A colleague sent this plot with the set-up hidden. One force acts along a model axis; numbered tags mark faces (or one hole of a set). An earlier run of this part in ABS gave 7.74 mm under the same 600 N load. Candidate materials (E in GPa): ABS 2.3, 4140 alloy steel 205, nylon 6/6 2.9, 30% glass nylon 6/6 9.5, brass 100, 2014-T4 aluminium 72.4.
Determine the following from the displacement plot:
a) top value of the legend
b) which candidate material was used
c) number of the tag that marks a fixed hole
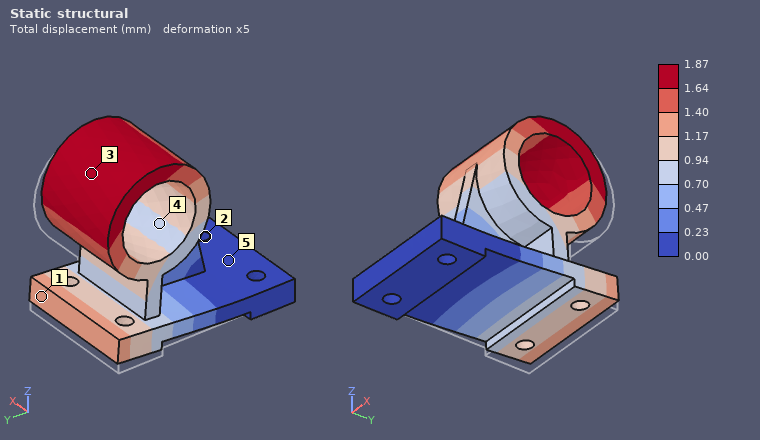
1.87 mm
30% glass nylon 6/6
2
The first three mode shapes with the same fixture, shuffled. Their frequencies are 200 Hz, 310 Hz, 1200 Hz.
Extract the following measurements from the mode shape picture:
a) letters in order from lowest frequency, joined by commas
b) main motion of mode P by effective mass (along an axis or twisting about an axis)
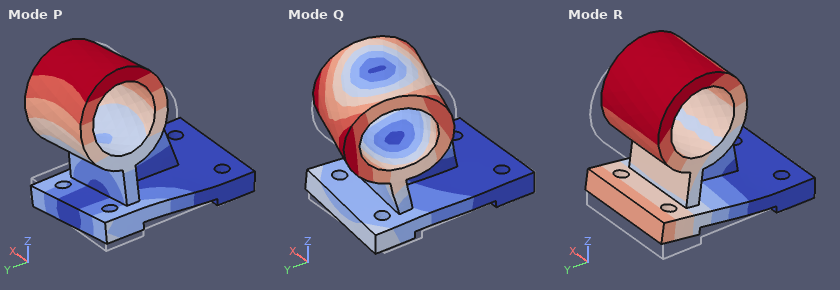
R, P, Q
along X
